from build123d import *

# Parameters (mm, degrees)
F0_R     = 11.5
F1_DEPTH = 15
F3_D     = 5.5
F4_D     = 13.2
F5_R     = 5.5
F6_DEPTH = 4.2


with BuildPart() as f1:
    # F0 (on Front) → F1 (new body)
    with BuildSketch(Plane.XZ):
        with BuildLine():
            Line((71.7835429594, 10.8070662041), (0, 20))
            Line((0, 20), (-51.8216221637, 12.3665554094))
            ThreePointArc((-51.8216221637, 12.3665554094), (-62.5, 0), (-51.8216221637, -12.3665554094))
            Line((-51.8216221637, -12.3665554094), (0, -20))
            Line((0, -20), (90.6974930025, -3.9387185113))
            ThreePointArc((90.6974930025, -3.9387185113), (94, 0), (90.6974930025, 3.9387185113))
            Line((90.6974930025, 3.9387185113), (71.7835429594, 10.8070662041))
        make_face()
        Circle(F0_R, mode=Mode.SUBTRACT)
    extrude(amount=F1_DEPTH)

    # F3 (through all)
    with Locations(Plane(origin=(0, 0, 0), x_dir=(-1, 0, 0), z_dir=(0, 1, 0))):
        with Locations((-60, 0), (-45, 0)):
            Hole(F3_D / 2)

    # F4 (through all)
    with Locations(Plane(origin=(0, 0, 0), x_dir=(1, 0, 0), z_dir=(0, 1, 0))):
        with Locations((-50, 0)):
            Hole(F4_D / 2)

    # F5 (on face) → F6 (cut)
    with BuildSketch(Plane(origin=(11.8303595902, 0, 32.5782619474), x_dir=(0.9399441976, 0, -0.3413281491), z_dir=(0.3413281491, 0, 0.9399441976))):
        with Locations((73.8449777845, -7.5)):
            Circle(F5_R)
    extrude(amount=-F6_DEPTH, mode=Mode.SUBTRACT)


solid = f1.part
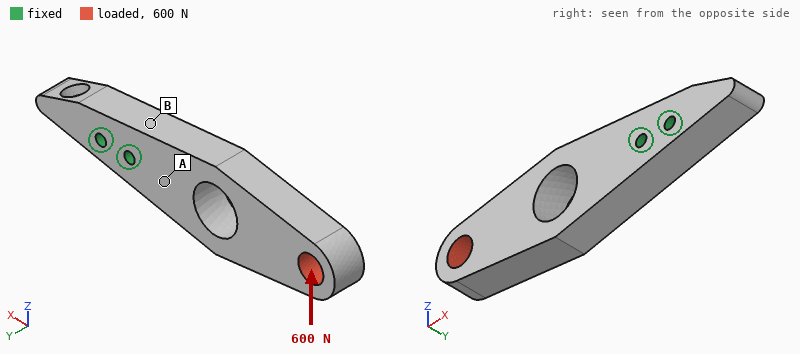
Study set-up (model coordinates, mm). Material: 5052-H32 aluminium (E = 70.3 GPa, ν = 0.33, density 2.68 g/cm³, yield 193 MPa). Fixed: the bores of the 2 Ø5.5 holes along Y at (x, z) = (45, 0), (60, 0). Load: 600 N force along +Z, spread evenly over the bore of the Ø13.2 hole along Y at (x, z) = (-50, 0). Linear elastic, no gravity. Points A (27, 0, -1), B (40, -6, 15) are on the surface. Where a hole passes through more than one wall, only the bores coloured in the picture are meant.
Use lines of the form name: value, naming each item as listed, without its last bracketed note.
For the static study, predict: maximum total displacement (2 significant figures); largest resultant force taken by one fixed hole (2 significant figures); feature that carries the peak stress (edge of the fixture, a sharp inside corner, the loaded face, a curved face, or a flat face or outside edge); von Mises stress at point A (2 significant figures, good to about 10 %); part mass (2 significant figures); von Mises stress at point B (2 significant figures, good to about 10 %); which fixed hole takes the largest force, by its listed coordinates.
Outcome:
maximum total displacement: 0.14 mm
largest resultant force taken by one fixed hole: 3.0 kN
feature that carries the peak stress: edge of the fixture
von Mises stress at point A: 7.4 MPa
part mass: 140 g
von Mises stress at point B: 29 MPa
which fixed hole takes the largest force, by its listed coordinates: (45, 0)
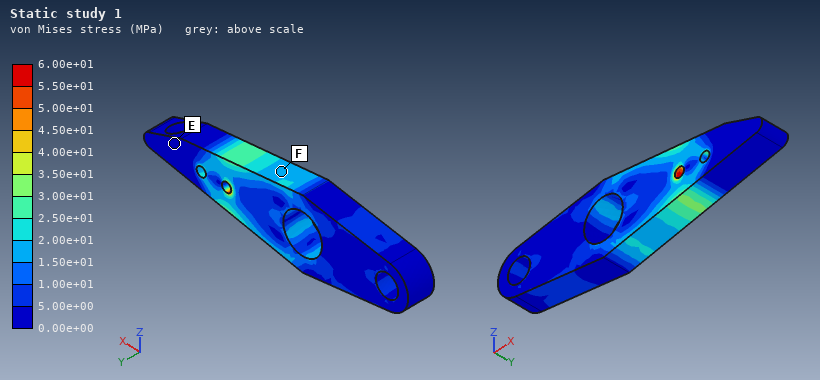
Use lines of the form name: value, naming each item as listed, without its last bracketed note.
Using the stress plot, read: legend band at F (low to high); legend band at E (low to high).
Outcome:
legend band at F: 1.50e+01 to 2.00e+01 MPa
legend band at E: 0.00e+00 to 5.00e+00 MPa
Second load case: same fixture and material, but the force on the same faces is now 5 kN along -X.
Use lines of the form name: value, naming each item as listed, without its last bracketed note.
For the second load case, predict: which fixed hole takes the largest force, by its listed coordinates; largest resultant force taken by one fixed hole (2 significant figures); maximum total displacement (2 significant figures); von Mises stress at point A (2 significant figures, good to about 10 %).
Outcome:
which fixed hole takes the largest force, by its listed coordinates: (45, 0)
largest resultant force taken by one fixed hole: 3.9 kN
maximum total displacement: 30 µm
von Mises stress at point A: 6.5 MPa
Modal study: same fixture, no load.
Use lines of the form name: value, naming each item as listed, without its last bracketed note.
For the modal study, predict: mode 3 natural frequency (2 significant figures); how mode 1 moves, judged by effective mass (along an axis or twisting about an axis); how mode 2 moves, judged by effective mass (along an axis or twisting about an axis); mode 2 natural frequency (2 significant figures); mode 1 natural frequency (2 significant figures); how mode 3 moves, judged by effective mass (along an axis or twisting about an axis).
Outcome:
mode 3 natural frequency: 5000 Hz
how mode 1 moves, judged by effective mass: along Y
how mode 2 moves, judged by effective mass: along Z
mode 2 natural frequency: 1800 Hz
mode 1 natural frequency: 1100 Hz
how mode 3 moves, judged by effective mass: twisting about X
